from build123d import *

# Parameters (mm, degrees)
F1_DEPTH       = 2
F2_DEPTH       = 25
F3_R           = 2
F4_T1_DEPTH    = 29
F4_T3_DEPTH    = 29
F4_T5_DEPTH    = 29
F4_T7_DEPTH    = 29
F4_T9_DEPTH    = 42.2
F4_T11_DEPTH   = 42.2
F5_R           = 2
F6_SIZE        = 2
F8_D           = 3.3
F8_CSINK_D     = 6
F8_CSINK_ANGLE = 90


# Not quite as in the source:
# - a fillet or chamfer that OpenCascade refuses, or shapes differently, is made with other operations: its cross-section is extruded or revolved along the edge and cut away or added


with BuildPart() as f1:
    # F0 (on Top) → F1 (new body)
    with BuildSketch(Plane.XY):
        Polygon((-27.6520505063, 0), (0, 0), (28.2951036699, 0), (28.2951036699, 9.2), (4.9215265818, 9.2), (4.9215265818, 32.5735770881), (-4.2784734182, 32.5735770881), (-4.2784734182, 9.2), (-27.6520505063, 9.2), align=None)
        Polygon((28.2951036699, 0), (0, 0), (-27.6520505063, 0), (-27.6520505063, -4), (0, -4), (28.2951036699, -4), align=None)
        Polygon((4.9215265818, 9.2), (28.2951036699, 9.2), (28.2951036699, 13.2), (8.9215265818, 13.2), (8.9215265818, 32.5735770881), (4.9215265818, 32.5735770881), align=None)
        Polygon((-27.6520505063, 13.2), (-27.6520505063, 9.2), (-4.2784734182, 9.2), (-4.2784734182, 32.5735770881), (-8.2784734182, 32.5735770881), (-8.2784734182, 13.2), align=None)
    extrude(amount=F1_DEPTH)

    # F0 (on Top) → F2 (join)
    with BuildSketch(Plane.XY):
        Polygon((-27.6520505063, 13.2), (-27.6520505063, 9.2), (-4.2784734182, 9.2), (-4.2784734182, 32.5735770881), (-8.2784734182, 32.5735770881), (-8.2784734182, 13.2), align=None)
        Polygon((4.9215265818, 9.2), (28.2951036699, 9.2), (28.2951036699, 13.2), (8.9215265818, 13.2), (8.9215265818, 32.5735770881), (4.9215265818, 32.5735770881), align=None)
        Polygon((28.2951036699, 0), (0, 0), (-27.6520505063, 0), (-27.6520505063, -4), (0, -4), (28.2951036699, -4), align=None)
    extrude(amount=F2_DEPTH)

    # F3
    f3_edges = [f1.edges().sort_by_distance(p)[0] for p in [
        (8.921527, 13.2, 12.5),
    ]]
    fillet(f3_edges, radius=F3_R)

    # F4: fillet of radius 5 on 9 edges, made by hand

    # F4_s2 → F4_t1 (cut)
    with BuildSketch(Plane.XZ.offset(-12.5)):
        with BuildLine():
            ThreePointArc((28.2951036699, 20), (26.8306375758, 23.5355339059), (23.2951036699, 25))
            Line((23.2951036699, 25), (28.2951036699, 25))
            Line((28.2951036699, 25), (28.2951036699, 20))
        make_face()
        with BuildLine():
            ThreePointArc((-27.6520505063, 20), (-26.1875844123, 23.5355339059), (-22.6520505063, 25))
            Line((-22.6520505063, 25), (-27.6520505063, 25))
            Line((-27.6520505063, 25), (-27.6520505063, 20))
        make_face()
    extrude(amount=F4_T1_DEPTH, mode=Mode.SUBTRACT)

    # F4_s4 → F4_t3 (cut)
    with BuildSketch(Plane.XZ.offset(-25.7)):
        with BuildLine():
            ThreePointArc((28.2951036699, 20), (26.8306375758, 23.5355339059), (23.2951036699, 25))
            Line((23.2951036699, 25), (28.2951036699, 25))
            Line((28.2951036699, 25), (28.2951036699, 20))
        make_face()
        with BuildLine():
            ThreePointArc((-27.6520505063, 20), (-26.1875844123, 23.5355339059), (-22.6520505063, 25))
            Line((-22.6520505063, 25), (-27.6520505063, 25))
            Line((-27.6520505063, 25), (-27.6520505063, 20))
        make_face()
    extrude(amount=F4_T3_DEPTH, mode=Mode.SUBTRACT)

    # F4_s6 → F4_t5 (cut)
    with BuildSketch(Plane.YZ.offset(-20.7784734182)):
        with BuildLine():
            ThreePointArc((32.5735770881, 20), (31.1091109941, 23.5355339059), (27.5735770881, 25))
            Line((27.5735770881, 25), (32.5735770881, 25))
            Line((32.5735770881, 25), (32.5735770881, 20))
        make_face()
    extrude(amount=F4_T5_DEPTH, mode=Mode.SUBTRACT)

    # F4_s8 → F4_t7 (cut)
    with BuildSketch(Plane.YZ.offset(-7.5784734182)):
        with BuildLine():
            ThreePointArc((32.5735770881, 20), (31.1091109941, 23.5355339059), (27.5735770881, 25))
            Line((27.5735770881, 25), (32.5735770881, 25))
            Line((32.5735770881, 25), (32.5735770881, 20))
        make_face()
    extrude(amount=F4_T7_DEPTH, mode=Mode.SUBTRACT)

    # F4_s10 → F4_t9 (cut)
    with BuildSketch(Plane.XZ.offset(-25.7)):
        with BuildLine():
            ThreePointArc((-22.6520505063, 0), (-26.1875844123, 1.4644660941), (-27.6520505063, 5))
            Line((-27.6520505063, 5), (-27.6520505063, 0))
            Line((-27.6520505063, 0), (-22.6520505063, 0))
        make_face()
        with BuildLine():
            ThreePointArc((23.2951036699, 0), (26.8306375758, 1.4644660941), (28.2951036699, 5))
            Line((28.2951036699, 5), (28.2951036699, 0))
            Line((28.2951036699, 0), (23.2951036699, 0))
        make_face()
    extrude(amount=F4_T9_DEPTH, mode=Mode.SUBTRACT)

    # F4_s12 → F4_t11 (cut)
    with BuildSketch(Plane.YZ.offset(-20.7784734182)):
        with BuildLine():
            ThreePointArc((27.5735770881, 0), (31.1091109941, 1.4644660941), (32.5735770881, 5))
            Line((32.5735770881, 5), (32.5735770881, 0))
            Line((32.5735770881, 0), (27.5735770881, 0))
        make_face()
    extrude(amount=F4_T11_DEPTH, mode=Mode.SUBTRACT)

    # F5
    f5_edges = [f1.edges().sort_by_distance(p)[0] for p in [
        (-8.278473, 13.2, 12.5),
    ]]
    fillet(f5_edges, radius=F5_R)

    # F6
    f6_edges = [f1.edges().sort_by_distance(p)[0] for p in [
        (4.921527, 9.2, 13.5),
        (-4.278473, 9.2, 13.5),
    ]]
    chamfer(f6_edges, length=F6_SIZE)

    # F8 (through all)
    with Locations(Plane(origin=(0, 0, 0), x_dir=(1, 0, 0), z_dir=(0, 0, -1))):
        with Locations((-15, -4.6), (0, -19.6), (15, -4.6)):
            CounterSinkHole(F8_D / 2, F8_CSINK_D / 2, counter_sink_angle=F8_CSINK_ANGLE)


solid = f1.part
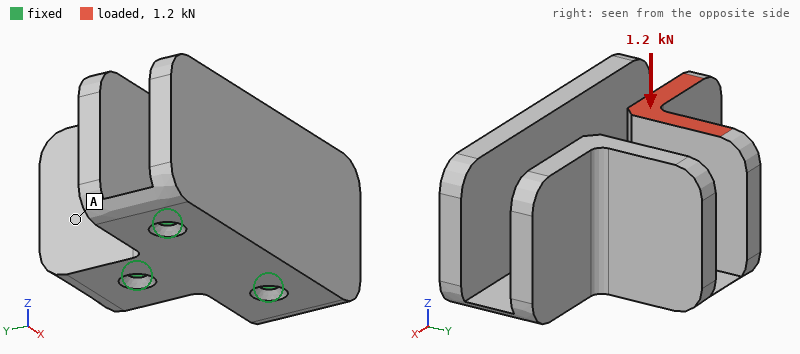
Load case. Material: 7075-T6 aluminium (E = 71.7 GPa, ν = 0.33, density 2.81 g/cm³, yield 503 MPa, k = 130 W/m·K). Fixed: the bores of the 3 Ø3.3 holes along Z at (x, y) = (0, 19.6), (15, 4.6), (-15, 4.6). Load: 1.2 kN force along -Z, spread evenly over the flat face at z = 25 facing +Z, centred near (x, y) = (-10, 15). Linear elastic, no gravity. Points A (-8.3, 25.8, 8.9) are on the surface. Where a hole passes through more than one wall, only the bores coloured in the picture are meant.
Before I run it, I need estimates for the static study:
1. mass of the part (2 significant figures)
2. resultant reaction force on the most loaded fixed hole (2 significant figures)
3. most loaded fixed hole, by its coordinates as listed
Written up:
42 g
730 N
(0, 19.6)
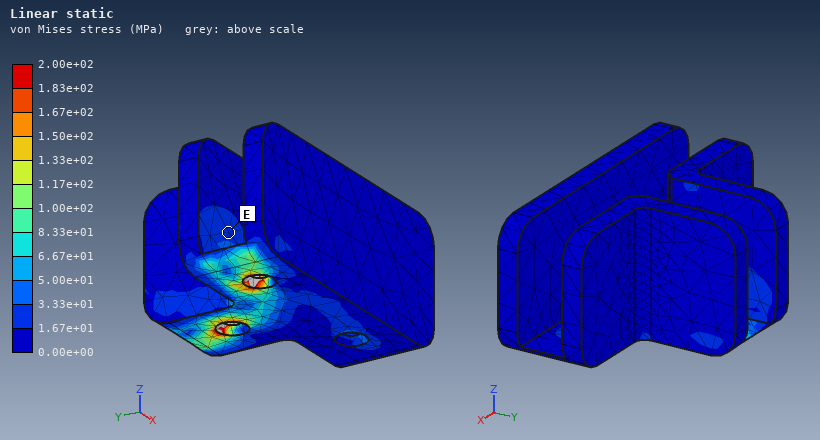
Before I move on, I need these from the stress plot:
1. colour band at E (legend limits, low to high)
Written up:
1.67e+01 to 3.33e+01 MPa
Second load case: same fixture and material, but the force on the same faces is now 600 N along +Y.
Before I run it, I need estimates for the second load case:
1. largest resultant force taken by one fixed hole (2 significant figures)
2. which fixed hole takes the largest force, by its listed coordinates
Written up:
990 N
(0, 19.6)
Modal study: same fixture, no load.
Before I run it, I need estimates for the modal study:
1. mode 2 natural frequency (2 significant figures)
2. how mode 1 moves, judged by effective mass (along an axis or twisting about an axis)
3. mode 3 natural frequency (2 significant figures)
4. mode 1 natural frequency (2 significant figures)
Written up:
2200 Hz
along Y
2600 Hz
1500 Hz
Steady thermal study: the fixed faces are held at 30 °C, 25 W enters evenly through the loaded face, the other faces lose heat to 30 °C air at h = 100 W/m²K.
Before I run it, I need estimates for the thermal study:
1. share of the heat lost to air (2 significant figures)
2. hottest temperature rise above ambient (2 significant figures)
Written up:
34 %
41 K
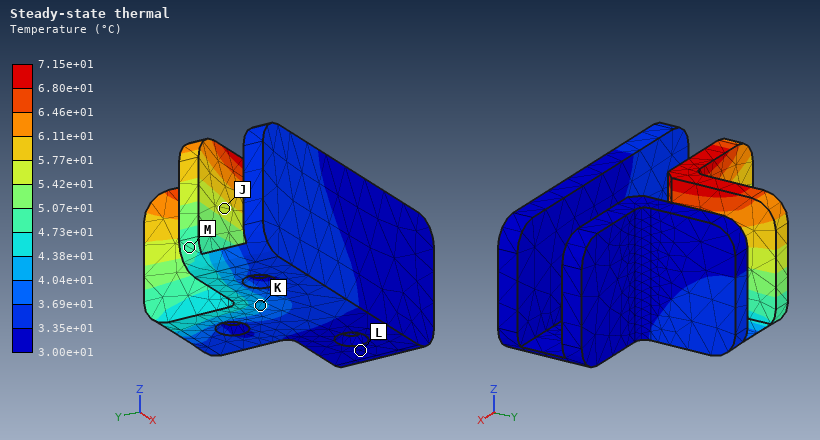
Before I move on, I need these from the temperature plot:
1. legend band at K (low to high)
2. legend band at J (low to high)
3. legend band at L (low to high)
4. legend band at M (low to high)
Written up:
4.04e+01 to 4.38e+01 °C
5.42e+01 to 5.77e+01 °C
3.00e+01 to 3.35e+01 °C
4.73e+01 to 5.07e+01 °C
